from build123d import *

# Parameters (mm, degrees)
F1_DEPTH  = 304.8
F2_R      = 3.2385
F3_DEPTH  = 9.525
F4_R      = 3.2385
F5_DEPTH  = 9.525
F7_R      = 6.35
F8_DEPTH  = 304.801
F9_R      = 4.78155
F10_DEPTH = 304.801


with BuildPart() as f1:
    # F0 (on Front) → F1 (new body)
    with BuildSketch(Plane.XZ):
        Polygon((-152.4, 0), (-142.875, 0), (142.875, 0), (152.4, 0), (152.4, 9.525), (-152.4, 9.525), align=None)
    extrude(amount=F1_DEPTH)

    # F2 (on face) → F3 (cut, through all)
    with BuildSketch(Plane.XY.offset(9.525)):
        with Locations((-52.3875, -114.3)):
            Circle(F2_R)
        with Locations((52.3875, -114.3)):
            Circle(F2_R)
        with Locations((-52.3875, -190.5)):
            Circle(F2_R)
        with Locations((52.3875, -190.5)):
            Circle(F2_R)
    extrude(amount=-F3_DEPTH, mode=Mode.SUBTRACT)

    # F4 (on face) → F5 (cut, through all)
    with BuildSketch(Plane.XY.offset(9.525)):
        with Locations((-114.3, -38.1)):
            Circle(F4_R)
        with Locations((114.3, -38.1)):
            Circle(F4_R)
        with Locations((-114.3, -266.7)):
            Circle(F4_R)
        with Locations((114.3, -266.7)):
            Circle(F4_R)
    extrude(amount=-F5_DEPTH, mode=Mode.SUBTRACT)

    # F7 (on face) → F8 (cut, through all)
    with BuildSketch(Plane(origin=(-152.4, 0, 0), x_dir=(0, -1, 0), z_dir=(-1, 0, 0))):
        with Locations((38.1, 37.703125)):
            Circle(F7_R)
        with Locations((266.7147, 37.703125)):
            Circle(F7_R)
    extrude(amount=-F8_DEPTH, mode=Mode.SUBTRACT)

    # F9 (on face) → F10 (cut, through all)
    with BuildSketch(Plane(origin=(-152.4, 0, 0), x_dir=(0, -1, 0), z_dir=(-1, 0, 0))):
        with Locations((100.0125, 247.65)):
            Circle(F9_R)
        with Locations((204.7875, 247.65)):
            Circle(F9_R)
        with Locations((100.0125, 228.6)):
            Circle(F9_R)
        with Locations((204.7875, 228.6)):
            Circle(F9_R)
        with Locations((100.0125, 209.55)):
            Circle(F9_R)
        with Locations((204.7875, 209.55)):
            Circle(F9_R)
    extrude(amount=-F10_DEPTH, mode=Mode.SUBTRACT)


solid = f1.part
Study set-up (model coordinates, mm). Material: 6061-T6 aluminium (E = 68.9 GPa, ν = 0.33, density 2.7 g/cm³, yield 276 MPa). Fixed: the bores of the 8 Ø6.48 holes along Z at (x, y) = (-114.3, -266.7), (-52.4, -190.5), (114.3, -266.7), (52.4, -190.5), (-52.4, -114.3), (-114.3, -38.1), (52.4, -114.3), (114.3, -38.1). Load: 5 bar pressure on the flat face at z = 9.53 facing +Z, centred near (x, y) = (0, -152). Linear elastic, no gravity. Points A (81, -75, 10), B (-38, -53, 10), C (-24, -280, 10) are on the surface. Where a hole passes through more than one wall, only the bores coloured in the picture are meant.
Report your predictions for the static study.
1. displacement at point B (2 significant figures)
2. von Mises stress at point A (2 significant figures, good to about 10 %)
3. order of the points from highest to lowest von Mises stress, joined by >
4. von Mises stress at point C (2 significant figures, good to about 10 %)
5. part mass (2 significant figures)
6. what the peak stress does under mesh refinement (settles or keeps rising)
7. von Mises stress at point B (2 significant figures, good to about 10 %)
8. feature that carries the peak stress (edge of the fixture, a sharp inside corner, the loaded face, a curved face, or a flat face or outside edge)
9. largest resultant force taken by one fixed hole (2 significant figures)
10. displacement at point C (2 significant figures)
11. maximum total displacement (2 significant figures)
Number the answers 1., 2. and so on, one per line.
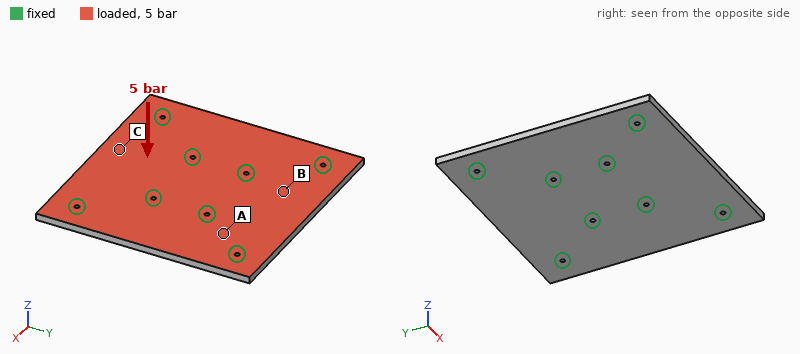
1. 0.25 mm
2. 55 MPa
3. A > C > B
4. 35 MPa
5. 2.4 kg
6. keeps rising
7. 24 MPa
8. edge of the fixture
9. 5.8 kN
10. 0.43 mm
11. 0.61 mm
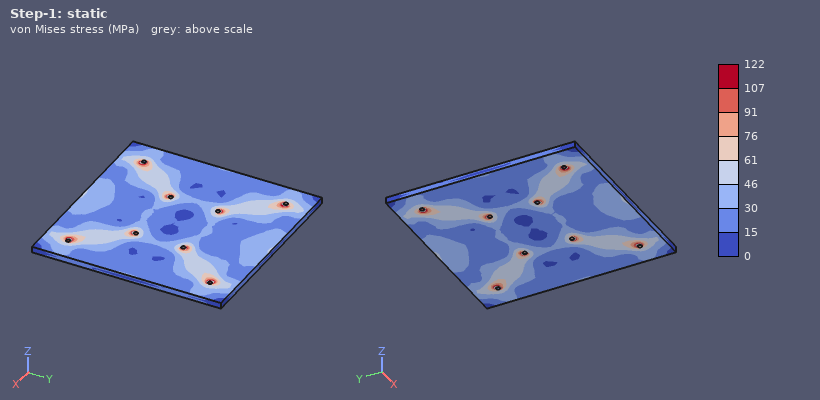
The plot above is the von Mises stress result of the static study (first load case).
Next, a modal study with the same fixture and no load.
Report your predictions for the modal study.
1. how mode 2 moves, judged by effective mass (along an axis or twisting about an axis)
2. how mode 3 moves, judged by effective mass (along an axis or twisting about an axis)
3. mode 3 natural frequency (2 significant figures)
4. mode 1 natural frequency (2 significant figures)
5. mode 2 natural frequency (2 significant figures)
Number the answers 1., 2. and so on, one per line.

1. twisting about X
2. twisting about Y
3. 1300 Hz
4. 1000 Hz
5. 1100 Hz
